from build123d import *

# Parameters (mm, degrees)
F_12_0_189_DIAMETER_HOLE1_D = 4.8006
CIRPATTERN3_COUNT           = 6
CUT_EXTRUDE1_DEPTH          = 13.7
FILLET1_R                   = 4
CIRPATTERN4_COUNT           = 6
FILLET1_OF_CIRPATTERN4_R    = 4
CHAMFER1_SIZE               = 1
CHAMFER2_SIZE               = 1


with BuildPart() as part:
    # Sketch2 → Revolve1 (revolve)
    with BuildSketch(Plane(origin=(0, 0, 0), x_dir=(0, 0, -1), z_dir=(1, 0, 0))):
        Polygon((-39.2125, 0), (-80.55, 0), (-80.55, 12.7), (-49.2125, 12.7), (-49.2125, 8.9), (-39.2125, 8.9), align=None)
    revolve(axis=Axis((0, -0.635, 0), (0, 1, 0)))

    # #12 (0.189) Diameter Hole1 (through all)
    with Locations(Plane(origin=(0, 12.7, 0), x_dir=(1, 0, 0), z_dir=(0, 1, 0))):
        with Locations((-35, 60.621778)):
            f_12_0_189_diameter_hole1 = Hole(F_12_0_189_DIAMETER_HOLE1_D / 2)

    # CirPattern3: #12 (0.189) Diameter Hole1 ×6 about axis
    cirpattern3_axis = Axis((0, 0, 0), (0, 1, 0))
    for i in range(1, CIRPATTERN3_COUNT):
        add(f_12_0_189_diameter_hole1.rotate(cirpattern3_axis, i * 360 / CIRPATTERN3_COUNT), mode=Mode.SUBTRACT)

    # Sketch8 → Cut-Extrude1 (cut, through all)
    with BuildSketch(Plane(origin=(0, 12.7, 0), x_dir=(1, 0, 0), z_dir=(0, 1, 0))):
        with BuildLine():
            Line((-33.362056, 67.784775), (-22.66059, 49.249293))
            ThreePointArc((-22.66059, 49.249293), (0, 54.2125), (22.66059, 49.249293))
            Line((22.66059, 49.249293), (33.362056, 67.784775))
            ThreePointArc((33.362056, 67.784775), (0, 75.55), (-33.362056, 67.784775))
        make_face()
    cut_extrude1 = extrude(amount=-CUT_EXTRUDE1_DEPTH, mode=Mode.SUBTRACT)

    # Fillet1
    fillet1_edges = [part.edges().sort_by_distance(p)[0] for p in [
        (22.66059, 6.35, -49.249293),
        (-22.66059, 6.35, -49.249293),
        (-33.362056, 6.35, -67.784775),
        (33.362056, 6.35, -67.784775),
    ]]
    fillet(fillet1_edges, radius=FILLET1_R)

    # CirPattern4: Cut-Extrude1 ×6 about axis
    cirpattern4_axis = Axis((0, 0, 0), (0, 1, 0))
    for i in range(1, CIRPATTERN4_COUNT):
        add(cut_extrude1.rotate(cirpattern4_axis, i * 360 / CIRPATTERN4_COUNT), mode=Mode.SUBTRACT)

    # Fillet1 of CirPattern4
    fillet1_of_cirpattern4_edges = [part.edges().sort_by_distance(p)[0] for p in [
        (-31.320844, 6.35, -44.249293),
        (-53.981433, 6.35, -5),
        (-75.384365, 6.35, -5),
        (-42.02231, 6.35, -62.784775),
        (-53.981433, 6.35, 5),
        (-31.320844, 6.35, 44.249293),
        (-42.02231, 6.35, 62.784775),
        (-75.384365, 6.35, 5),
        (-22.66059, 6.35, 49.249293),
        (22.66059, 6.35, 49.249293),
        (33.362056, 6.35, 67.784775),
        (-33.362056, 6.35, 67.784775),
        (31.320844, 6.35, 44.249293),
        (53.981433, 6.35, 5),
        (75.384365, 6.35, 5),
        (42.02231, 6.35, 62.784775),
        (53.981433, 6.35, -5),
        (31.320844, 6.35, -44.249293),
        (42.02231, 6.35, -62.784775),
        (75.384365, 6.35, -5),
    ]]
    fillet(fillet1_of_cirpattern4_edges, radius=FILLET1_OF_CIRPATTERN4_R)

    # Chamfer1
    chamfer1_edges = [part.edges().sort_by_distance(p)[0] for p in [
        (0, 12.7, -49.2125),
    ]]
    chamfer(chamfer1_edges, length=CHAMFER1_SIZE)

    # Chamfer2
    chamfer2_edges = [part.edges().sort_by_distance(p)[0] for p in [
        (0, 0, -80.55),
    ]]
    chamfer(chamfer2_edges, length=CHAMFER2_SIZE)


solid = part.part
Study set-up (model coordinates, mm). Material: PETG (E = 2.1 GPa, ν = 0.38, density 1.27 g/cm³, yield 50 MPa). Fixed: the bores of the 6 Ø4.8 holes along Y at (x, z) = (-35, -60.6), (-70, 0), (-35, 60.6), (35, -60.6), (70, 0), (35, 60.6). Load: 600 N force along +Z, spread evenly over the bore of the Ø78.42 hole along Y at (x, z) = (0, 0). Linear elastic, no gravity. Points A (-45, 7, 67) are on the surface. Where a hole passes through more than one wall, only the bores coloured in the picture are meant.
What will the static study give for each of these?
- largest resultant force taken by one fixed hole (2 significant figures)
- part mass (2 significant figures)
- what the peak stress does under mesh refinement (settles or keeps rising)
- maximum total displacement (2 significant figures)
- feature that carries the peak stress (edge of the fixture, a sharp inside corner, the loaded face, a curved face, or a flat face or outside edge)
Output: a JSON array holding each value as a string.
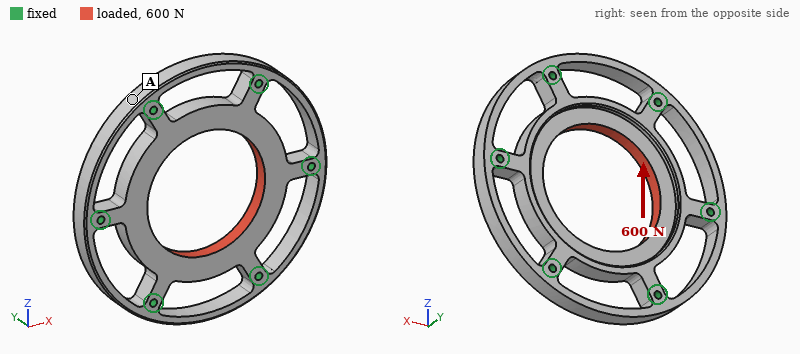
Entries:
["140 N", "120 g", "keeps rising", "35 µm", "edge of the fixture"]
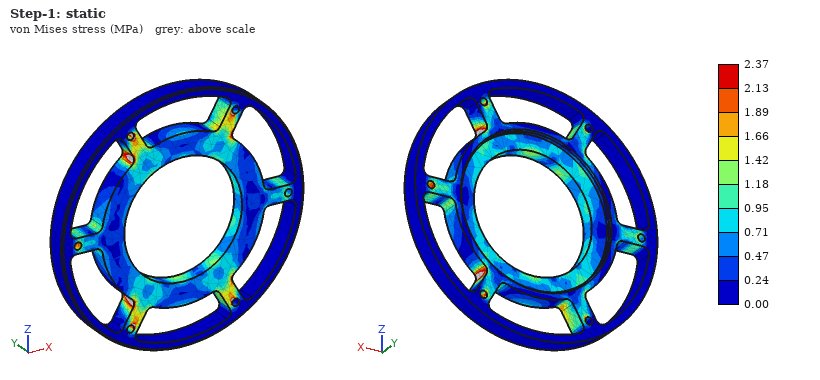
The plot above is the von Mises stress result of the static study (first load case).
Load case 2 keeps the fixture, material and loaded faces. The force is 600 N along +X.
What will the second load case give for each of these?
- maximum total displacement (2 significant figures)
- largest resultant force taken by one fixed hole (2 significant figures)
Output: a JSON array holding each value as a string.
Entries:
["32 µm", "160 N"]
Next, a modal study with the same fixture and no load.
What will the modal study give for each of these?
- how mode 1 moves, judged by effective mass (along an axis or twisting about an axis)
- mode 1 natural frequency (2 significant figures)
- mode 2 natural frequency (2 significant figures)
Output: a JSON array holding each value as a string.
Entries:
["along Y", "1600 Hz", "1800 Hz"]
